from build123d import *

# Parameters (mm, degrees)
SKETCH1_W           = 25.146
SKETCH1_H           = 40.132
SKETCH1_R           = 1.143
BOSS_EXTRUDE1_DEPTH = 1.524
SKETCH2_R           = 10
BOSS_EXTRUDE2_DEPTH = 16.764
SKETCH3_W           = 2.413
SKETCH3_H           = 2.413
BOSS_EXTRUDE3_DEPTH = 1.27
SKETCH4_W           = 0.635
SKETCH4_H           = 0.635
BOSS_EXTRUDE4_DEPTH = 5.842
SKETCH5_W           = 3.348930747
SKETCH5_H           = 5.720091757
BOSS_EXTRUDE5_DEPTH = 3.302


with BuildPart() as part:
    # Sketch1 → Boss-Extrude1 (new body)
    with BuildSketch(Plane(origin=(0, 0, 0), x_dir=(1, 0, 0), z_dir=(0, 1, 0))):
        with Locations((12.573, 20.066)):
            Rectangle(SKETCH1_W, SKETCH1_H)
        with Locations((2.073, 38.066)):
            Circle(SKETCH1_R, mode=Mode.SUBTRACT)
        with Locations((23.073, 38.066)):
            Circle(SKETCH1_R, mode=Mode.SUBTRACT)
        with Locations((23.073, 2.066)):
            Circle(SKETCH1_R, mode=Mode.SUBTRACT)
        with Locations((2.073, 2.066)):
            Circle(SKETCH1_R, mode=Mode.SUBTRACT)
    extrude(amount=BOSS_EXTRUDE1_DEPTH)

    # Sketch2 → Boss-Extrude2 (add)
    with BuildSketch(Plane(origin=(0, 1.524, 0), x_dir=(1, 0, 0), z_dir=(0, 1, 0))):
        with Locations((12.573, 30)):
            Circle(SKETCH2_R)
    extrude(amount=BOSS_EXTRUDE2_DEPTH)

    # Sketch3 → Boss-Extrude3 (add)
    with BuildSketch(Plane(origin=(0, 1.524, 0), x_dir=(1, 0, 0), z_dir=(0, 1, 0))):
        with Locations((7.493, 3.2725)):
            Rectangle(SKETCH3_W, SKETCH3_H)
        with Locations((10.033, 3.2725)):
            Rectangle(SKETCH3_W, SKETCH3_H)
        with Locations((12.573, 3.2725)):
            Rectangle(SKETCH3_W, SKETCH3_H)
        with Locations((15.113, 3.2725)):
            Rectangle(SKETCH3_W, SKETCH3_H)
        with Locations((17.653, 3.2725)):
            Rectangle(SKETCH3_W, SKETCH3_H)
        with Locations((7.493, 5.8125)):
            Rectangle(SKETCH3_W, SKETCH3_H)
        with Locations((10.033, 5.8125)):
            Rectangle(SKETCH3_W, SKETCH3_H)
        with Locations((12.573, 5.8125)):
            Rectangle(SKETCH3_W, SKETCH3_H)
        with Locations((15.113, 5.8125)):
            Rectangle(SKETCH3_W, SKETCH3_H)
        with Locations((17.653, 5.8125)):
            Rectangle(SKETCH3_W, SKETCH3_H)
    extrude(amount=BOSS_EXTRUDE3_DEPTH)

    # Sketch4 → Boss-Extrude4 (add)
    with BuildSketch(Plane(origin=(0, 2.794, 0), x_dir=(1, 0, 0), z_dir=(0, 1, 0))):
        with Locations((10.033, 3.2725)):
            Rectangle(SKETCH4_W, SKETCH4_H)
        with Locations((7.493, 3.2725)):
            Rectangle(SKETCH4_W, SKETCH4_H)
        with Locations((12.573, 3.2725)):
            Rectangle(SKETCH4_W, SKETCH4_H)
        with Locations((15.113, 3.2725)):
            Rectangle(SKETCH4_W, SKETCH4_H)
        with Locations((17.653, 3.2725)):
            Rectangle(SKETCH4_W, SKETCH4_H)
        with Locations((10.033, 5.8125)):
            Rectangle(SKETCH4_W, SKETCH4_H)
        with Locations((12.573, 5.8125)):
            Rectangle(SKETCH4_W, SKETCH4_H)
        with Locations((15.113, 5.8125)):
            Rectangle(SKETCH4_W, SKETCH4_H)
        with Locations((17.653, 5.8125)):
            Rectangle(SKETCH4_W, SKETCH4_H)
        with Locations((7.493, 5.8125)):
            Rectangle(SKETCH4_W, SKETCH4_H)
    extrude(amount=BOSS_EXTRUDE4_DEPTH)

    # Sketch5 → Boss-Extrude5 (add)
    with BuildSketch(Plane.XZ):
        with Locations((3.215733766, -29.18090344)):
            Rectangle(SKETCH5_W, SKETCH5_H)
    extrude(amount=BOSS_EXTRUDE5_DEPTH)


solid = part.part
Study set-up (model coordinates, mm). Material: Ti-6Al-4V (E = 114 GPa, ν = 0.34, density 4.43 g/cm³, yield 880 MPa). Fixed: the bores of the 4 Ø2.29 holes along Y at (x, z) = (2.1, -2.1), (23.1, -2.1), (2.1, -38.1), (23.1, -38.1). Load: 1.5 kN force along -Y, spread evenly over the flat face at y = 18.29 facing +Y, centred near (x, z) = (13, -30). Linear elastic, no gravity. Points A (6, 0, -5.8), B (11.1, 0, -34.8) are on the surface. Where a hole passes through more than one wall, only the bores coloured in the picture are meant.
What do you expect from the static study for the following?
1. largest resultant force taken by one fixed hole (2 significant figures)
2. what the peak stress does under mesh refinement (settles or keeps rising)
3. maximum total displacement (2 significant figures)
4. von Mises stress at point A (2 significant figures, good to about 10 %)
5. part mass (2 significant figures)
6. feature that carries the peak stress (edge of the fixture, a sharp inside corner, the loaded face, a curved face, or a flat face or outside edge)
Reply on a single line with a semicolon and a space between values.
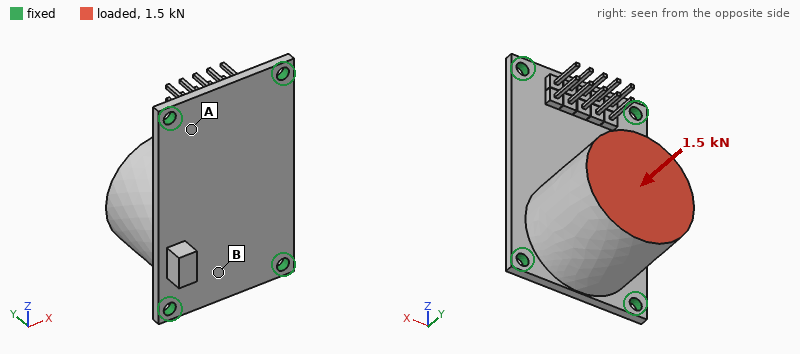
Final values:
640 N; keeps rising; 0.23 mm; 99 MPa; 31 g; edge of the fixture
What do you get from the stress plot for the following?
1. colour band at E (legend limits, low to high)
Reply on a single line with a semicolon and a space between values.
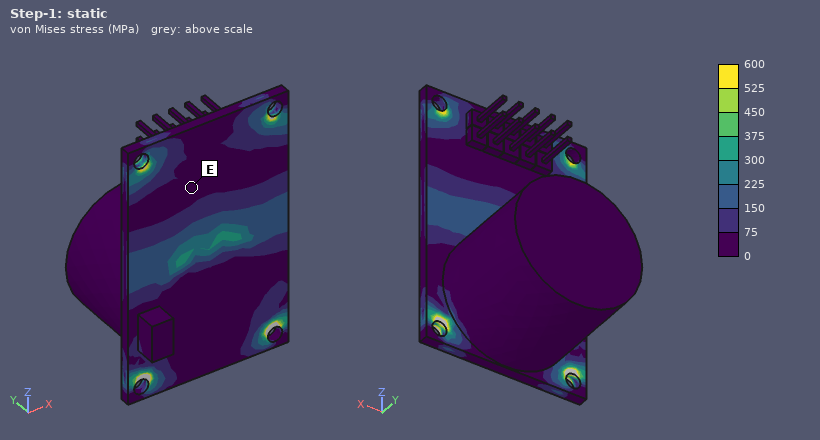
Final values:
0 to 75 MPa
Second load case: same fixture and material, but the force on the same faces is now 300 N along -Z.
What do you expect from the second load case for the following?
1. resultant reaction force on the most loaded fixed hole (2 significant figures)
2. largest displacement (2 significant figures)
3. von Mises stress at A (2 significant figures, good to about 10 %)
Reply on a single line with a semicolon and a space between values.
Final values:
140 N; 0.12 mm; 50 MPa
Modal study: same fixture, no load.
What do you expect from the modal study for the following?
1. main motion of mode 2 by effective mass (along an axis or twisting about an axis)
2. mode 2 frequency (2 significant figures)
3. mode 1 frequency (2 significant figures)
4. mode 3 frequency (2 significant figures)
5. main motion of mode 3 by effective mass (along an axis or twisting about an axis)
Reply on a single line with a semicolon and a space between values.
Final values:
along X; 6900 Hz; 2300 Hz; 10000 Hz; along Y
